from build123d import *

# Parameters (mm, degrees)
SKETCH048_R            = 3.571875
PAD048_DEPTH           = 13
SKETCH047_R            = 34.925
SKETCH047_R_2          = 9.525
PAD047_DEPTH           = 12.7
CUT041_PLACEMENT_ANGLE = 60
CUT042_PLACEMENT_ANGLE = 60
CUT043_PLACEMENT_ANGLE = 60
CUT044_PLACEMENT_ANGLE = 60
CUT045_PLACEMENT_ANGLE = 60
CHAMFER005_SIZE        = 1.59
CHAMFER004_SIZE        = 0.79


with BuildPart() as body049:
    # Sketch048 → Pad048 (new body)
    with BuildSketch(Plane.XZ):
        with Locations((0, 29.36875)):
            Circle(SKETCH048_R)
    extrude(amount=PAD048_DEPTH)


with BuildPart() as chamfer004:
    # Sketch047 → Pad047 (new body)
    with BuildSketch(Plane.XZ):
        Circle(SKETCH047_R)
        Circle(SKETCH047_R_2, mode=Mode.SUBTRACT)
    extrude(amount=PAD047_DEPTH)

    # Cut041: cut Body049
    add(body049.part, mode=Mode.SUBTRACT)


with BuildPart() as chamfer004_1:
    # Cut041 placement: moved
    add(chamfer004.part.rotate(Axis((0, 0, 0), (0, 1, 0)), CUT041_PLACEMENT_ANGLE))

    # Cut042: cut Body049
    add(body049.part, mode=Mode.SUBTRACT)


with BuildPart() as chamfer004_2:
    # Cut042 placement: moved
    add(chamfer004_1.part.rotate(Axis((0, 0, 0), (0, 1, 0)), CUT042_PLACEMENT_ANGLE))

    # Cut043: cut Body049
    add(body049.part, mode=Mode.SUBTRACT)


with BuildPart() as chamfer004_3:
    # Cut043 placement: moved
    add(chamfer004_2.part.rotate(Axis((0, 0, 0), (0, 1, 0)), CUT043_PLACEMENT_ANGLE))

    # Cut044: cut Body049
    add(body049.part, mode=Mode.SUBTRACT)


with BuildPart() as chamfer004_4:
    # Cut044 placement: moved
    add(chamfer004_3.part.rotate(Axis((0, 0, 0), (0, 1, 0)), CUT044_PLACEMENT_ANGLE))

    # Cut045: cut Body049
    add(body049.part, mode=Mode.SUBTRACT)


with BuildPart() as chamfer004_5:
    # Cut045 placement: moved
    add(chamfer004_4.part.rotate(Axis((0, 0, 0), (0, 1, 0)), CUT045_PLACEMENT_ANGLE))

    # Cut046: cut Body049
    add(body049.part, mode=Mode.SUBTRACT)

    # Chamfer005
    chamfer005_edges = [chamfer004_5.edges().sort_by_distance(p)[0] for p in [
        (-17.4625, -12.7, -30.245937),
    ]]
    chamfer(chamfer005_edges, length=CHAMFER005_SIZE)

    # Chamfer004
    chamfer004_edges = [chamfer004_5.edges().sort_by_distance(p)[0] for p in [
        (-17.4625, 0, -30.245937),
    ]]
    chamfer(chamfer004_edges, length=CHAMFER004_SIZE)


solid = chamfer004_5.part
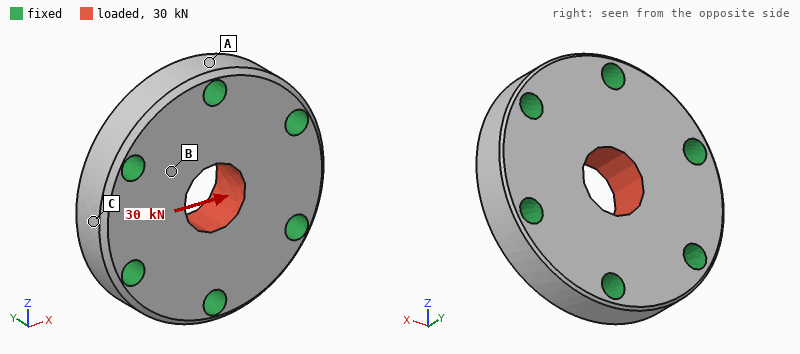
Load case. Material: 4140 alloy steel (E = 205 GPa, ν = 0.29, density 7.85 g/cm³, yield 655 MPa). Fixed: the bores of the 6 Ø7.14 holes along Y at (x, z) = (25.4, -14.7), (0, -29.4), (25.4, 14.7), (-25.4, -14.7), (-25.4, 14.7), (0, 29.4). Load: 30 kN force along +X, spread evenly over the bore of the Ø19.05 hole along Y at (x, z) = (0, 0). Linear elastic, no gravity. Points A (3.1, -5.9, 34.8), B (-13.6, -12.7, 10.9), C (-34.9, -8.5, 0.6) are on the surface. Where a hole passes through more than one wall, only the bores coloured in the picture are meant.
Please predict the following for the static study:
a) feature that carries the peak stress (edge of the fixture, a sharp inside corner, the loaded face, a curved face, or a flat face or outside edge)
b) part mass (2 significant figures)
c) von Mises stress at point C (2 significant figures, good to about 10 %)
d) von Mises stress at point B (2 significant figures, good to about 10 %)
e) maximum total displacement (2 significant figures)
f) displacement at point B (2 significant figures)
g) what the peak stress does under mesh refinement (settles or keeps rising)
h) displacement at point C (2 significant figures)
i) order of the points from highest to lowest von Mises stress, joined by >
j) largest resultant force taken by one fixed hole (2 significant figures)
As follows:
edge of the fixture
330 g
18 MPa
37 MPa
3.7 µm
1.7 µm
keeps rising
1.4 µm
B > C > A
6.8 kN
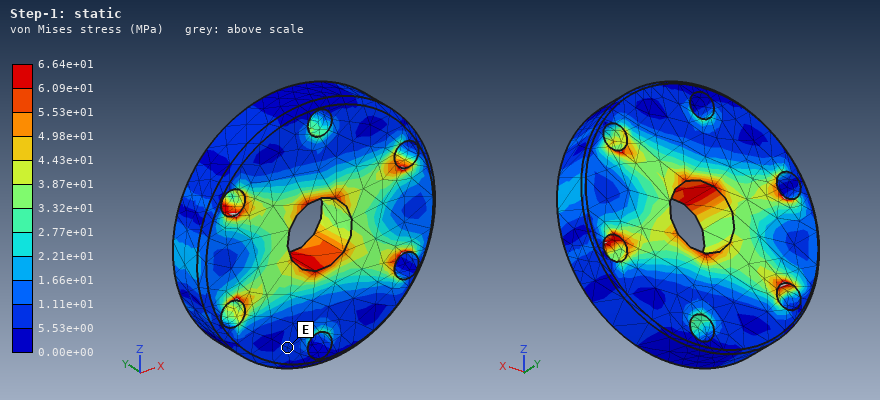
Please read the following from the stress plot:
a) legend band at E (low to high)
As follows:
5.53e+00 to 1.11e+01 MPa
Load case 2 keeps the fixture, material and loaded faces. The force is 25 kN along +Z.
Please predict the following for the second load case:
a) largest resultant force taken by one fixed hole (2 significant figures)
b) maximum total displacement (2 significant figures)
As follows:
6.4 kN
3.1 µm
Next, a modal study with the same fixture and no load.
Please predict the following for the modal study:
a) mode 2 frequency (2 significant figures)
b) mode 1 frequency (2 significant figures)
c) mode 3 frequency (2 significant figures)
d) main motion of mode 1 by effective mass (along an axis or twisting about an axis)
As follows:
39 kHz
28 kHz
39 kHz
along Y
